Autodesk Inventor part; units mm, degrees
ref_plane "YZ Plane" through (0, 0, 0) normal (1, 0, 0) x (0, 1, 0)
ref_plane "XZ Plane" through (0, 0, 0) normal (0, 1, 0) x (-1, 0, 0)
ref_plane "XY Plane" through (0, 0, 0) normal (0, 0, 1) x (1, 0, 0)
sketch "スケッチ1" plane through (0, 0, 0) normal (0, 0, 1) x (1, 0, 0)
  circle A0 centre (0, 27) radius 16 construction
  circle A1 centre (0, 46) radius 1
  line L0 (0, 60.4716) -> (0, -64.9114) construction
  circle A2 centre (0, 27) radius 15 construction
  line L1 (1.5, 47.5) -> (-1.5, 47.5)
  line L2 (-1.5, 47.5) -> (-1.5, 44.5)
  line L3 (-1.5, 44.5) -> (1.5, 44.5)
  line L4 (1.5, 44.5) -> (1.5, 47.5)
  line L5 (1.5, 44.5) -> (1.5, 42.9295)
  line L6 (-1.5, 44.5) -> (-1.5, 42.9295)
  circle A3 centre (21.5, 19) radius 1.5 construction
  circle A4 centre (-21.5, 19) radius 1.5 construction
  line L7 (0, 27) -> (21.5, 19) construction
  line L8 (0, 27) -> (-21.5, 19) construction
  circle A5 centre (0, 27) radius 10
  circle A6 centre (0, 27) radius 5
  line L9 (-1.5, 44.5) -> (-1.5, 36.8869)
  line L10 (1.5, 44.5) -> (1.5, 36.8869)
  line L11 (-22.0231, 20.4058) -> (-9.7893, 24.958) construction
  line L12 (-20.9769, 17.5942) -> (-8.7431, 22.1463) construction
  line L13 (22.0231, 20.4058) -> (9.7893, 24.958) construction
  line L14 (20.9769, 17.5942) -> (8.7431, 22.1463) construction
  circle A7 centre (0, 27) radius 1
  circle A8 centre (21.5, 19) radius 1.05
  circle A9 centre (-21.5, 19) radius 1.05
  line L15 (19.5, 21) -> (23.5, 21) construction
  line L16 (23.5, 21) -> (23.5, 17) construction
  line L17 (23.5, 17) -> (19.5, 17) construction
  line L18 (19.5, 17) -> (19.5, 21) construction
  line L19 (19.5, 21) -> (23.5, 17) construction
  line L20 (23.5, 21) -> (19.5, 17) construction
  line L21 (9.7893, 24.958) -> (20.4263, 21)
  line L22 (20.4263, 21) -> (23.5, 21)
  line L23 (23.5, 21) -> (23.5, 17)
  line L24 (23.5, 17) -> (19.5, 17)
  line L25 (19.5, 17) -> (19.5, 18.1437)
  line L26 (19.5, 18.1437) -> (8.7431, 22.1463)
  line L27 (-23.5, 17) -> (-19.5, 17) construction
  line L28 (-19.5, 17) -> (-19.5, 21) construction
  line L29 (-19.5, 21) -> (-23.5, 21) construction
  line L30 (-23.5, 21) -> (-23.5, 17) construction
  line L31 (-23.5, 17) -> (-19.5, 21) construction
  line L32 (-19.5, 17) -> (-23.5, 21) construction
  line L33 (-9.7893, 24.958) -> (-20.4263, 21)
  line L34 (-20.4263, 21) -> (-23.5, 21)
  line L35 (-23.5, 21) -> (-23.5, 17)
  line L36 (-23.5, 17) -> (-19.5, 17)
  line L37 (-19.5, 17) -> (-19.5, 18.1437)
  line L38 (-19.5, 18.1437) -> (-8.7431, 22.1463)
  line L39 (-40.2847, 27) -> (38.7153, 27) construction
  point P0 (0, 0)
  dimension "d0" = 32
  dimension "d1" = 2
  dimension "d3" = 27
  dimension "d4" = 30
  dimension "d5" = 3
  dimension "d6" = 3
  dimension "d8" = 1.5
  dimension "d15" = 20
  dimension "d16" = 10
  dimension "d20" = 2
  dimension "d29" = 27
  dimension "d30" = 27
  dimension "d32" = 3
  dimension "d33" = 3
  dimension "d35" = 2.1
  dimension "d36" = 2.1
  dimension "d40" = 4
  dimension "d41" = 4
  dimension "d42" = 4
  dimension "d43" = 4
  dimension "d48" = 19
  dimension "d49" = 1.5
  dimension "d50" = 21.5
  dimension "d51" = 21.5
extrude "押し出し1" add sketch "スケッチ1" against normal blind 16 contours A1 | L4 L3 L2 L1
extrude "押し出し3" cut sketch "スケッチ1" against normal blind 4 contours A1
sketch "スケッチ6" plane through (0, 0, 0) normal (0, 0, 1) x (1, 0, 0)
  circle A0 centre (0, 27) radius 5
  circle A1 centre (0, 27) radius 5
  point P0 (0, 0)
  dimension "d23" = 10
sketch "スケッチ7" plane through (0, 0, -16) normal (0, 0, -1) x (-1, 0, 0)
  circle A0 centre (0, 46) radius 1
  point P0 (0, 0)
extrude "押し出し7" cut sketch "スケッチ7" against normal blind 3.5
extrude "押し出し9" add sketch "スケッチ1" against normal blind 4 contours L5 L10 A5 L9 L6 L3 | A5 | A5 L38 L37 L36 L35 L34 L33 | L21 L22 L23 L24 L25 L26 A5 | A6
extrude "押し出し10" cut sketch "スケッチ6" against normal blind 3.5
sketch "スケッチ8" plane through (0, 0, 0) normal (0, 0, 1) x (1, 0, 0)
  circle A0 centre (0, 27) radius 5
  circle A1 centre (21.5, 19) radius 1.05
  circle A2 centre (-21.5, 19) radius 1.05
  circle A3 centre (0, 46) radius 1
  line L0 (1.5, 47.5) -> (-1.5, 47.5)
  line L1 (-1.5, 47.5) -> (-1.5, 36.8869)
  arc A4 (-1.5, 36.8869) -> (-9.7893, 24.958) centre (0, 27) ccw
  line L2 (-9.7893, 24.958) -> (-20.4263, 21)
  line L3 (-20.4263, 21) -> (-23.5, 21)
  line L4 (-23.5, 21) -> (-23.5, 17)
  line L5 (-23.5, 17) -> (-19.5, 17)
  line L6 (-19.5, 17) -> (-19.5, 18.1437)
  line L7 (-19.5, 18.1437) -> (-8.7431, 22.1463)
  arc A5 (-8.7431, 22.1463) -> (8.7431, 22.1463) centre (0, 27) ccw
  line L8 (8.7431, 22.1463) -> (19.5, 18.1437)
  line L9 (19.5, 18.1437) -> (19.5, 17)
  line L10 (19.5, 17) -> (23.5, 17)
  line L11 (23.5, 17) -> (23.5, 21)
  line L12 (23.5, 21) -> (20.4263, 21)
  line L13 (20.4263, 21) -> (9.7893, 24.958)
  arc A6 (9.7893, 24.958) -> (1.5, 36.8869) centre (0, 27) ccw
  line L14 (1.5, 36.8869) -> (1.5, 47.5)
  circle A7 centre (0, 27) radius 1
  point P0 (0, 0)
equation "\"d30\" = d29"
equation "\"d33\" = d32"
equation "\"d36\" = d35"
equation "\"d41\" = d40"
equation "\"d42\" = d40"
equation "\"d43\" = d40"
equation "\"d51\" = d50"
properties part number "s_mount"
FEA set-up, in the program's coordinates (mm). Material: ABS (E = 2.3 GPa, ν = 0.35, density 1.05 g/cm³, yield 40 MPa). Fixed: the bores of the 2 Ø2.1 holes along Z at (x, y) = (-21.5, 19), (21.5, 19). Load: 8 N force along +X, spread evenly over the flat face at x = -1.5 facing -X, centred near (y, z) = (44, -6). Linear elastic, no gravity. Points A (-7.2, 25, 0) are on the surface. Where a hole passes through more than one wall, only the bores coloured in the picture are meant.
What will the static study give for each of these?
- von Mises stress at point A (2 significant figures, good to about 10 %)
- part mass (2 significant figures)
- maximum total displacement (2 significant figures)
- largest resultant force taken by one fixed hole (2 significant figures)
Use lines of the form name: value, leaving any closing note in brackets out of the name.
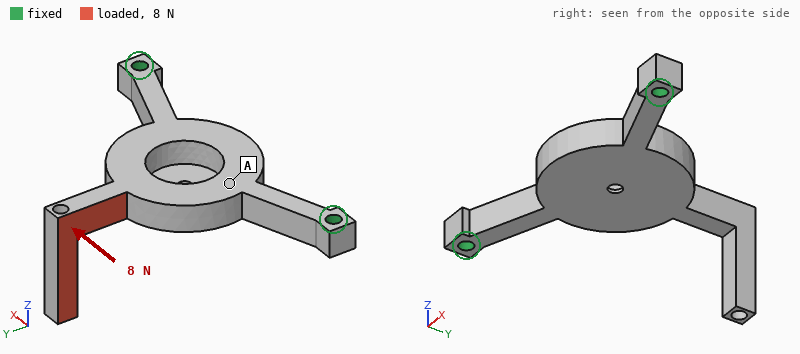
von Mises stress at point A: 1.0 MPa
part mass: 1.6 g
maximum total displacement: 0.54 mm
largest resultant force taken by one fixed hole: 7.1 N
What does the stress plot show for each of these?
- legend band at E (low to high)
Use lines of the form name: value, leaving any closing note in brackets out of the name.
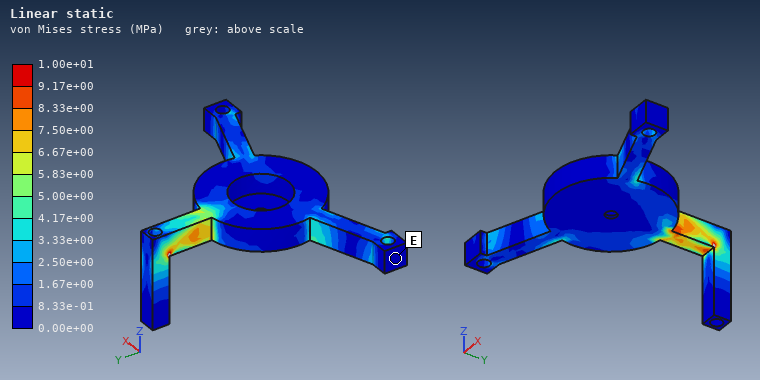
legend band at E: 0.00e+00 to 8.33e-01 MPa
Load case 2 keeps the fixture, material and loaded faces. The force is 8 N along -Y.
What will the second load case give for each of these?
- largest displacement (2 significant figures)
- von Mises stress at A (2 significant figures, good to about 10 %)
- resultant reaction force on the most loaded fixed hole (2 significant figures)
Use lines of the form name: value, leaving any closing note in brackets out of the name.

largest displacement: 0.56 mm
von Mises stress at A: 0.87 MPa
resultant reaction force on the most loaded fixed hole: 8.3 N
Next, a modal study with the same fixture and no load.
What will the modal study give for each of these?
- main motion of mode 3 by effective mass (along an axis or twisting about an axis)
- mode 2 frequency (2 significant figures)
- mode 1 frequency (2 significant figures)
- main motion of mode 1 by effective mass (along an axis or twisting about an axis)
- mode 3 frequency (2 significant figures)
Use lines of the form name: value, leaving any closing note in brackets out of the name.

main motion of mode 3 by effective mass: along Z
mode 2 frequency: 1700 Hz
mode 1 frequency: 610 Hz
main motion of mode 1 by effective mass: along Z
mode 3 frequency: 2200 Hz
